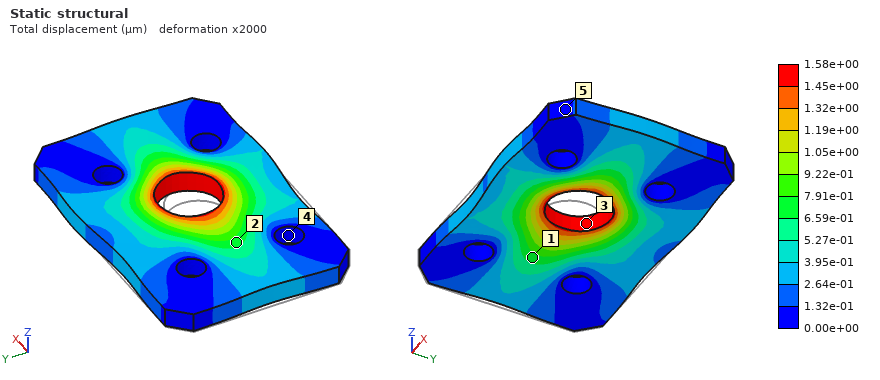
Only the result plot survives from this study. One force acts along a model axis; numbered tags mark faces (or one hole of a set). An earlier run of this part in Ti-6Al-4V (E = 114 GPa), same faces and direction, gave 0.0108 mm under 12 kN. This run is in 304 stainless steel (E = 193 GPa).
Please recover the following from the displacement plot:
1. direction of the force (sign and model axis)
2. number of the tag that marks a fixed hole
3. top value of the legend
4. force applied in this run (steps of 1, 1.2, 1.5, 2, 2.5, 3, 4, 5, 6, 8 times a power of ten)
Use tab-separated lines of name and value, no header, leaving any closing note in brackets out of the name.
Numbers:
direction of the force	+X
number of the tag that marks a fixed hole	4
top value of the legend	1.58e+00 µm
force applied in this run	3 kN
